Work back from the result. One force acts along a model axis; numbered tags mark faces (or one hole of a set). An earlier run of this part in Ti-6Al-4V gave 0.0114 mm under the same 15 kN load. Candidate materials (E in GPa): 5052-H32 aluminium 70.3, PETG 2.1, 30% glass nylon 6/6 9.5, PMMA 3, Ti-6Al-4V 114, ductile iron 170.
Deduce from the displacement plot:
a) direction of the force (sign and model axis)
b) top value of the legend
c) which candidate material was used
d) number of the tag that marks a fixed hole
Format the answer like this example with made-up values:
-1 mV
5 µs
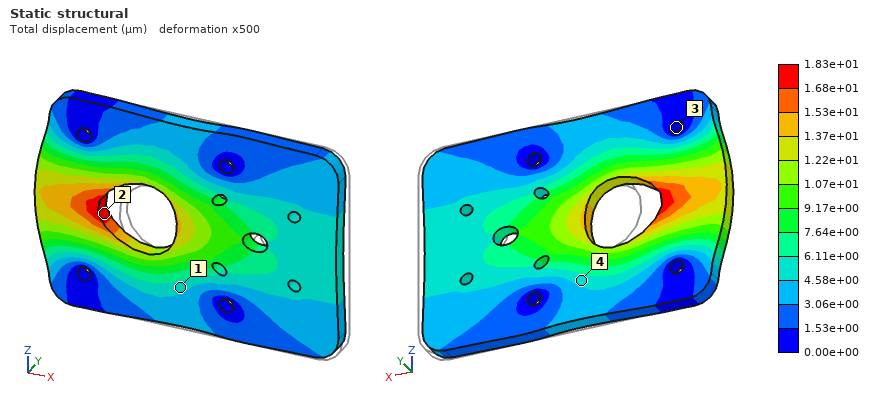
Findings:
-X
1.83e+01 µm
5052-H32 aluminium
3
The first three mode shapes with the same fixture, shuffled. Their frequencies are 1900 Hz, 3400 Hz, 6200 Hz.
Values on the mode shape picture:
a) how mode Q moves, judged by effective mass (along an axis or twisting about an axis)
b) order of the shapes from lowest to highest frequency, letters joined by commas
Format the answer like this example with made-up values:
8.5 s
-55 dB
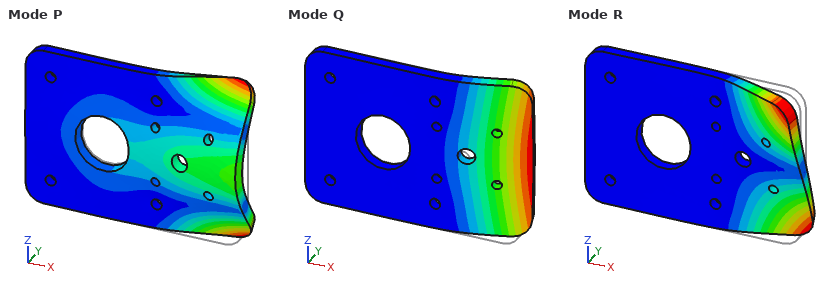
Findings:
along Y
Q, R, P
